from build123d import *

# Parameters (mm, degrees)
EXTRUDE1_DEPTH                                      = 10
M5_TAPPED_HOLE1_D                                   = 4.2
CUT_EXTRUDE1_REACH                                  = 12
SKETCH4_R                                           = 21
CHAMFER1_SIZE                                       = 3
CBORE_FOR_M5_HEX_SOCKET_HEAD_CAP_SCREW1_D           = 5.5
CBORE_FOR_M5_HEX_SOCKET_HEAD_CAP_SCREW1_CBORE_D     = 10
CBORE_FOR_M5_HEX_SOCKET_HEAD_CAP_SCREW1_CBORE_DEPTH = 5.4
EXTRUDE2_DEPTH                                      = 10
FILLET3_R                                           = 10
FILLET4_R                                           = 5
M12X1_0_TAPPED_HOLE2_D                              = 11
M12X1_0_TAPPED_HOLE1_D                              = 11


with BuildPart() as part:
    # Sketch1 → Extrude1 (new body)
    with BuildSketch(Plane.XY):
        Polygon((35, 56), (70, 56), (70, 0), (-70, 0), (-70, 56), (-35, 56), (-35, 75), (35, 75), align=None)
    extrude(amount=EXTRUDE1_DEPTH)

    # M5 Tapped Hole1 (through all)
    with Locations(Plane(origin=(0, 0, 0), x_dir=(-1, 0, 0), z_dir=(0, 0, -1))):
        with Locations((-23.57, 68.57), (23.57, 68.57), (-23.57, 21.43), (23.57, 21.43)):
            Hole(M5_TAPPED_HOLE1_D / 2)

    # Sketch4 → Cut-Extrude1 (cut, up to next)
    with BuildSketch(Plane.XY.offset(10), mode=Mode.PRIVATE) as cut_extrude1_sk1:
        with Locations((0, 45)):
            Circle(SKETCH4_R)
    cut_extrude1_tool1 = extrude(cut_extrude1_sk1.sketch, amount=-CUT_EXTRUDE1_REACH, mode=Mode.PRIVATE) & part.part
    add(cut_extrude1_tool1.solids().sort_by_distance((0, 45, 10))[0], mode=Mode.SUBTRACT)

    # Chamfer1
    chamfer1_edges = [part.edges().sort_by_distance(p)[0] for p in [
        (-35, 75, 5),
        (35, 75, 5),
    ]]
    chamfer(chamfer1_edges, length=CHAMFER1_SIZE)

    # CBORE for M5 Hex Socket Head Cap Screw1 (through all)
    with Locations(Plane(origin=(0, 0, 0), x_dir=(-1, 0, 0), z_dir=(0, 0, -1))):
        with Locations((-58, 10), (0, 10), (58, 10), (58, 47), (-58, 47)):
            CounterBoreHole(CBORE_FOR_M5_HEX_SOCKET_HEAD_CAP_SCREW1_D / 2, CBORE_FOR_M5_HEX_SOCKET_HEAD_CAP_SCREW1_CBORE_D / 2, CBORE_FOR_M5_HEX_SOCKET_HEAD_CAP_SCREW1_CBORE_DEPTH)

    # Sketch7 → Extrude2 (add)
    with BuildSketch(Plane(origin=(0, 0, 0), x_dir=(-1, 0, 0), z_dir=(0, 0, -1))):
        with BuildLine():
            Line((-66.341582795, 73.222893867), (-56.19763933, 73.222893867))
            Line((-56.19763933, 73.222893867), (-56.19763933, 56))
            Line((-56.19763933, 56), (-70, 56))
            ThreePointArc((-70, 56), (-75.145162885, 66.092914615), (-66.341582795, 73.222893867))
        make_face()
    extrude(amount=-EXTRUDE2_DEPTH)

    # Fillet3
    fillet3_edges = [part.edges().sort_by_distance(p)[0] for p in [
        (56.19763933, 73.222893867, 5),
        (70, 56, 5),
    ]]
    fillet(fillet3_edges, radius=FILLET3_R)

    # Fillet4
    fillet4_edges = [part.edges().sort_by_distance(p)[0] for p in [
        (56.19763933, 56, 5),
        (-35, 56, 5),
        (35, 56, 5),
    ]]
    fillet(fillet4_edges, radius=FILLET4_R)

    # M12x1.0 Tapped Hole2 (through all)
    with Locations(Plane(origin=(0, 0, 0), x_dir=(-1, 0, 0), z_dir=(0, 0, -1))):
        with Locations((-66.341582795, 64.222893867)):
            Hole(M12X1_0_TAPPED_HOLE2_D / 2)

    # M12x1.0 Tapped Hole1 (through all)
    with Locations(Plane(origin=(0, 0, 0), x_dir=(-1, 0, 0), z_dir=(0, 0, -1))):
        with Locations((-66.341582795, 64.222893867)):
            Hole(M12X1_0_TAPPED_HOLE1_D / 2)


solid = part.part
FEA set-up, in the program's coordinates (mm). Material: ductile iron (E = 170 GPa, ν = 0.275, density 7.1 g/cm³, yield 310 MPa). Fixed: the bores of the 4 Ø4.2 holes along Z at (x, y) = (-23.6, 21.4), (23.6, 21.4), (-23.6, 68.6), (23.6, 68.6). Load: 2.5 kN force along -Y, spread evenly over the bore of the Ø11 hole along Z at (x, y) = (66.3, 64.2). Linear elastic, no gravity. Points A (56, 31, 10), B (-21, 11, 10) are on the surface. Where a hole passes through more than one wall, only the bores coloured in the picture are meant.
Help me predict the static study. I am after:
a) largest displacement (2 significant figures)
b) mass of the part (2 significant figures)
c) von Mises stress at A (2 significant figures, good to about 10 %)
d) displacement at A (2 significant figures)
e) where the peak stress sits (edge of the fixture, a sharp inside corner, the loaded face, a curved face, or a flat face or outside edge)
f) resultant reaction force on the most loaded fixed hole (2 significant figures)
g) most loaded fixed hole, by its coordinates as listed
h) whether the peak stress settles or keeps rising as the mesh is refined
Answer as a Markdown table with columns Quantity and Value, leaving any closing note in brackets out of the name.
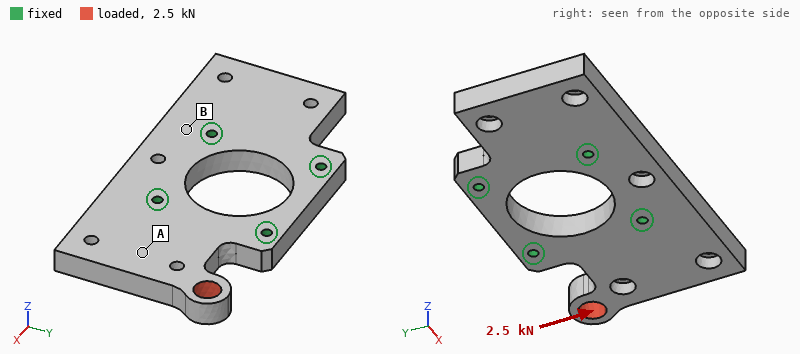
| Quantity | Value |
|---|---|
| largest displacement | 28 µm |
| mass of the part | 540 g |
| von Mises stress at A | 13 MPa |
| displacement at A | 6.2 µm |
| where the peak stress sits | a sharp inside corner |
| resultant reaction force on the most loaded fixed hole | 2.4 kN |
| most loaded fixed hole, by its coordinates as listed | (23.6, 68.6) |
| whether the peak stress settles or keeps rising as the mesh is refined | keeps rising |
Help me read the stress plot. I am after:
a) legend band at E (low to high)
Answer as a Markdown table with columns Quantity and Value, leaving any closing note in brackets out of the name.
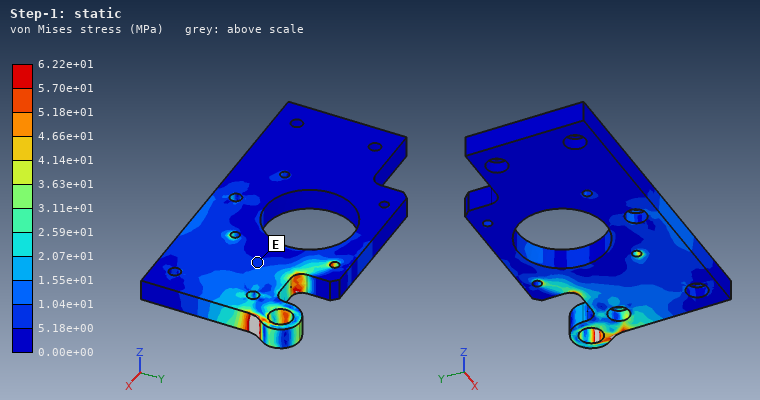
| Quantity | Value |
|---|---|
| legend band at E | 5.18e+00 to 1.04e+01 MPa |
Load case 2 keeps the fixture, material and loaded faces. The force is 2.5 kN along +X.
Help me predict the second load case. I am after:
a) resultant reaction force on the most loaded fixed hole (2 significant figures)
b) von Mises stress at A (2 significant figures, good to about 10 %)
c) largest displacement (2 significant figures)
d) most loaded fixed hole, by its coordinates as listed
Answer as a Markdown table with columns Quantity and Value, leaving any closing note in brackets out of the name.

| Quantity | Value |
|---|---|
| resultant reaction force on the most loaded fixed hole | 2.3 kN |
| von Mises stress at A | 10.0 MPa |
| largest displacement | 44 µm |
| most loaded fixed hole, by its coordinates as listed | (23.6, 68.6) |
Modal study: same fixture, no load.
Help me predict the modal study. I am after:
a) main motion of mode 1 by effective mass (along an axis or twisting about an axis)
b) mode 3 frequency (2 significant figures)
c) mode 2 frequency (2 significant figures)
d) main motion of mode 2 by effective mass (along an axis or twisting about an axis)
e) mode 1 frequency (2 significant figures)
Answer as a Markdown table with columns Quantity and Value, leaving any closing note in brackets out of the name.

| Quantity | Value |
|---|---|
| main motion of mode 1 by effective mass | along Z |
| mode 3 frequency | 4800 Hz |
| mode 2 frequency | 3000 Hz |
| main motion of mode 2 by effective mass | along Z |
| mode 1 frequency | 2700 Hz |
